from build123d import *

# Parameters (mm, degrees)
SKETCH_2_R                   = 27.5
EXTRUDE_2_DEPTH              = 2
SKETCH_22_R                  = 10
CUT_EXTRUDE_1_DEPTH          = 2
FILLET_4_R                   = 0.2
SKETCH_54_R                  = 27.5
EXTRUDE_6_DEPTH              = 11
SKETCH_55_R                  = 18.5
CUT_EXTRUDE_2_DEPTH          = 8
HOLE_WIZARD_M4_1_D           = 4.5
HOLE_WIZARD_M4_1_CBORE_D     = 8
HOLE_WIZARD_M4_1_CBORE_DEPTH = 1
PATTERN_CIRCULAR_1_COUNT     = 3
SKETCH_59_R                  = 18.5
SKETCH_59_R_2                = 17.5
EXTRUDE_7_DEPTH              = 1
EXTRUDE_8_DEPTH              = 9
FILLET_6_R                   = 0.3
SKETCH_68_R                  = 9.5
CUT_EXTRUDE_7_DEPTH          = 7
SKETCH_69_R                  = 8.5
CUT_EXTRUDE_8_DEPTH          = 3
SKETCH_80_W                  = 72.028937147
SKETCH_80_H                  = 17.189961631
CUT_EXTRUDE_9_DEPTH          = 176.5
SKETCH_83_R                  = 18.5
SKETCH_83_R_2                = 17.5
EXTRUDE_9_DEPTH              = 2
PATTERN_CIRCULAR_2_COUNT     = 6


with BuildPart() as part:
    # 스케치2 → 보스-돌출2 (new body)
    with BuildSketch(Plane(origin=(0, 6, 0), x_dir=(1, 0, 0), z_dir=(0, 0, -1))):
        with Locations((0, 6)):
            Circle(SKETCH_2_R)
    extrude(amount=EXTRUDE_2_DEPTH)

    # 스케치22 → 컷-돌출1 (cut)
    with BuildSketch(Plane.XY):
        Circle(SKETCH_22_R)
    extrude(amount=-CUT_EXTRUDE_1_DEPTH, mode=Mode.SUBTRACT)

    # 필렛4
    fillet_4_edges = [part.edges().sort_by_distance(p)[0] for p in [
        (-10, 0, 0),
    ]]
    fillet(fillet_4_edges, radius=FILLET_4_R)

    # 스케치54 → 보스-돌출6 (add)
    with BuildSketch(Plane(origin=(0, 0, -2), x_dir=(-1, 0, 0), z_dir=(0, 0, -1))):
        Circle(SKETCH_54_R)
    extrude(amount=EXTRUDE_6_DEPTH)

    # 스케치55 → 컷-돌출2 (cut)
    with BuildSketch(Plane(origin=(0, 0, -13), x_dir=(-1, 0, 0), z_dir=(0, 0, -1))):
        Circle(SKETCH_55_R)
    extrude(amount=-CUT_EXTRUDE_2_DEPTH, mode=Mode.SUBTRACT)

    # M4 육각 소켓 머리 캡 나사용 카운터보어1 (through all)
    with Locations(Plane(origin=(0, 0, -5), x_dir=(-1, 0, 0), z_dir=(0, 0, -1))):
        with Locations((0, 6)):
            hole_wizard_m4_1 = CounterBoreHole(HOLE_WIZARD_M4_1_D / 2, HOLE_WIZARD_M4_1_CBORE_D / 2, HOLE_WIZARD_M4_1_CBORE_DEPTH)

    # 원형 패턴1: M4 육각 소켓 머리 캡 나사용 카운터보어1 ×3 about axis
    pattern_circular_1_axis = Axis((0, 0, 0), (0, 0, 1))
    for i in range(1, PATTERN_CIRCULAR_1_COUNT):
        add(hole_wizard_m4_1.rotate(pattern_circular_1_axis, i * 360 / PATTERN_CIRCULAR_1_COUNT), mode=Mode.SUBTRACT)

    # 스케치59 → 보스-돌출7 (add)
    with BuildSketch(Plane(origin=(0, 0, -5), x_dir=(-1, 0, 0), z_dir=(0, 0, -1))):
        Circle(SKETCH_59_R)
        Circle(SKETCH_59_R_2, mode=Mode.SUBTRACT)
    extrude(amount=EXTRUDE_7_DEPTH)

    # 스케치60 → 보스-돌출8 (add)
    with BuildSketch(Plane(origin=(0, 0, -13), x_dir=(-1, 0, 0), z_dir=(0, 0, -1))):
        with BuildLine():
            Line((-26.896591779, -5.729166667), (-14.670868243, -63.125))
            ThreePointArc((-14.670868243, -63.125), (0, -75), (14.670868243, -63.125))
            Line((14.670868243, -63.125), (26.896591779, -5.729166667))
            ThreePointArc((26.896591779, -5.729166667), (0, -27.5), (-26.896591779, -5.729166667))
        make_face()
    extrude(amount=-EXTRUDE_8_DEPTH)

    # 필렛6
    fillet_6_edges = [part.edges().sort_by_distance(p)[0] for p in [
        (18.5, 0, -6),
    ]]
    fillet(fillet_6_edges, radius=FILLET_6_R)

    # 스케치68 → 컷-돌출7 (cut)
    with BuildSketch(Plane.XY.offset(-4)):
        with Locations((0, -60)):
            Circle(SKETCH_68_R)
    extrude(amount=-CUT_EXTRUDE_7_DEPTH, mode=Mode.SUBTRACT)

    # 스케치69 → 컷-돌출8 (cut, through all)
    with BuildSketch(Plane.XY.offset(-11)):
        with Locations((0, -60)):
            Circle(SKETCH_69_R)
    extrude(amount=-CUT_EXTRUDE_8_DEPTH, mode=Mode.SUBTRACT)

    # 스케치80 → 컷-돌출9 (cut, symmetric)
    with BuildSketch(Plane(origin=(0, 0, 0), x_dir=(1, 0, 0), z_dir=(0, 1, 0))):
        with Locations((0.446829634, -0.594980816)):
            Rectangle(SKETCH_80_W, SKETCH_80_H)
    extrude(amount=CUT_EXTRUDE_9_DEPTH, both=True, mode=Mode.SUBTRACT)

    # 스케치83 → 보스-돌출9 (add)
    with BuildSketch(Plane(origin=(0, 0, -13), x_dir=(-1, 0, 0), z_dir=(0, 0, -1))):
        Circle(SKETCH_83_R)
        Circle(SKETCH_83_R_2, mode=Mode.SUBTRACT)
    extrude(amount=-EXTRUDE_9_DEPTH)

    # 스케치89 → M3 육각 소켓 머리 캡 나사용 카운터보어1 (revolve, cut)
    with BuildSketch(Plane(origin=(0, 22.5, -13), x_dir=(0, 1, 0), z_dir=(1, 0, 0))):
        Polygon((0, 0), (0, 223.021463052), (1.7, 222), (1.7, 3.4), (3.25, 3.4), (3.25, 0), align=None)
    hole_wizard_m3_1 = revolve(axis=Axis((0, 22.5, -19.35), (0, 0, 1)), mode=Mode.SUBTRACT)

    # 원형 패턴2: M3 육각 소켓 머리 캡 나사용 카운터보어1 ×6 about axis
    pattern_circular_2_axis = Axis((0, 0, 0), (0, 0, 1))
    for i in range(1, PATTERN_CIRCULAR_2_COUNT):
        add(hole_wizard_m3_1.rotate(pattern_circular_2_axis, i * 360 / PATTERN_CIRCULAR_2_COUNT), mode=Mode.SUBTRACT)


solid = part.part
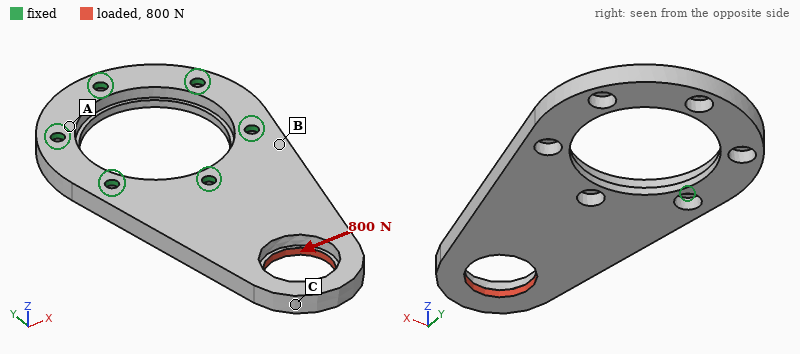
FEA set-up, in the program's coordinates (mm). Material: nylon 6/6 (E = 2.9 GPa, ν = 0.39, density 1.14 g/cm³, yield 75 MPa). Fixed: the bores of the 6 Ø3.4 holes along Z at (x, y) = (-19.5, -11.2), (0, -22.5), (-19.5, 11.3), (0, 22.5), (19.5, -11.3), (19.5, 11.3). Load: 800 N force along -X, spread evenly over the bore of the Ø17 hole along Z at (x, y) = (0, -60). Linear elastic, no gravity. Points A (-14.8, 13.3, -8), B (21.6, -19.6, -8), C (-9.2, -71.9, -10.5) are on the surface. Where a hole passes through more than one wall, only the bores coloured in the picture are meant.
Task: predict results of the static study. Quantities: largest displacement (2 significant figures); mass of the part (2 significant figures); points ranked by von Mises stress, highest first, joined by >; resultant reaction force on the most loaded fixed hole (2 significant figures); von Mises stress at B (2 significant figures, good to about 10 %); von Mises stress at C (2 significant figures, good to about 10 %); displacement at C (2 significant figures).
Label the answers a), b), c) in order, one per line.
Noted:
a) 1.1 mm
b) 15 g
c) B > C > A
d) 710 N
e) 27 MPa
f) 16 MPa
g) 1.0 mm
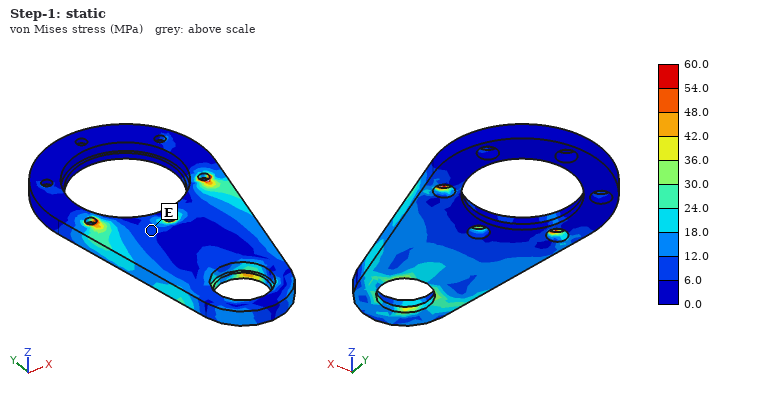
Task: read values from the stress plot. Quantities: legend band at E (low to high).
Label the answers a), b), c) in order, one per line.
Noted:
a) 6.0 to 12.0 MPa
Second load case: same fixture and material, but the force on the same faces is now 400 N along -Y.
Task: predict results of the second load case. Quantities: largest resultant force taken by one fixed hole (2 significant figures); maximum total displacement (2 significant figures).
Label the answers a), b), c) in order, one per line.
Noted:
a) 140 N
b) 1.2 mm
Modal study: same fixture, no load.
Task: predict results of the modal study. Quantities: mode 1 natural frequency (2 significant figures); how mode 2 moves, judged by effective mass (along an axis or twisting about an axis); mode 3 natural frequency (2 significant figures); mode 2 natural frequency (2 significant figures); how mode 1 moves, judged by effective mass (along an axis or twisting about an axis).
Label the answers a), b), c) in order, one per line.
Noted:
a) 520 Hz
b) twisting about Y
c) 2100 Hz
d) 1400 Hz
e) along Z
